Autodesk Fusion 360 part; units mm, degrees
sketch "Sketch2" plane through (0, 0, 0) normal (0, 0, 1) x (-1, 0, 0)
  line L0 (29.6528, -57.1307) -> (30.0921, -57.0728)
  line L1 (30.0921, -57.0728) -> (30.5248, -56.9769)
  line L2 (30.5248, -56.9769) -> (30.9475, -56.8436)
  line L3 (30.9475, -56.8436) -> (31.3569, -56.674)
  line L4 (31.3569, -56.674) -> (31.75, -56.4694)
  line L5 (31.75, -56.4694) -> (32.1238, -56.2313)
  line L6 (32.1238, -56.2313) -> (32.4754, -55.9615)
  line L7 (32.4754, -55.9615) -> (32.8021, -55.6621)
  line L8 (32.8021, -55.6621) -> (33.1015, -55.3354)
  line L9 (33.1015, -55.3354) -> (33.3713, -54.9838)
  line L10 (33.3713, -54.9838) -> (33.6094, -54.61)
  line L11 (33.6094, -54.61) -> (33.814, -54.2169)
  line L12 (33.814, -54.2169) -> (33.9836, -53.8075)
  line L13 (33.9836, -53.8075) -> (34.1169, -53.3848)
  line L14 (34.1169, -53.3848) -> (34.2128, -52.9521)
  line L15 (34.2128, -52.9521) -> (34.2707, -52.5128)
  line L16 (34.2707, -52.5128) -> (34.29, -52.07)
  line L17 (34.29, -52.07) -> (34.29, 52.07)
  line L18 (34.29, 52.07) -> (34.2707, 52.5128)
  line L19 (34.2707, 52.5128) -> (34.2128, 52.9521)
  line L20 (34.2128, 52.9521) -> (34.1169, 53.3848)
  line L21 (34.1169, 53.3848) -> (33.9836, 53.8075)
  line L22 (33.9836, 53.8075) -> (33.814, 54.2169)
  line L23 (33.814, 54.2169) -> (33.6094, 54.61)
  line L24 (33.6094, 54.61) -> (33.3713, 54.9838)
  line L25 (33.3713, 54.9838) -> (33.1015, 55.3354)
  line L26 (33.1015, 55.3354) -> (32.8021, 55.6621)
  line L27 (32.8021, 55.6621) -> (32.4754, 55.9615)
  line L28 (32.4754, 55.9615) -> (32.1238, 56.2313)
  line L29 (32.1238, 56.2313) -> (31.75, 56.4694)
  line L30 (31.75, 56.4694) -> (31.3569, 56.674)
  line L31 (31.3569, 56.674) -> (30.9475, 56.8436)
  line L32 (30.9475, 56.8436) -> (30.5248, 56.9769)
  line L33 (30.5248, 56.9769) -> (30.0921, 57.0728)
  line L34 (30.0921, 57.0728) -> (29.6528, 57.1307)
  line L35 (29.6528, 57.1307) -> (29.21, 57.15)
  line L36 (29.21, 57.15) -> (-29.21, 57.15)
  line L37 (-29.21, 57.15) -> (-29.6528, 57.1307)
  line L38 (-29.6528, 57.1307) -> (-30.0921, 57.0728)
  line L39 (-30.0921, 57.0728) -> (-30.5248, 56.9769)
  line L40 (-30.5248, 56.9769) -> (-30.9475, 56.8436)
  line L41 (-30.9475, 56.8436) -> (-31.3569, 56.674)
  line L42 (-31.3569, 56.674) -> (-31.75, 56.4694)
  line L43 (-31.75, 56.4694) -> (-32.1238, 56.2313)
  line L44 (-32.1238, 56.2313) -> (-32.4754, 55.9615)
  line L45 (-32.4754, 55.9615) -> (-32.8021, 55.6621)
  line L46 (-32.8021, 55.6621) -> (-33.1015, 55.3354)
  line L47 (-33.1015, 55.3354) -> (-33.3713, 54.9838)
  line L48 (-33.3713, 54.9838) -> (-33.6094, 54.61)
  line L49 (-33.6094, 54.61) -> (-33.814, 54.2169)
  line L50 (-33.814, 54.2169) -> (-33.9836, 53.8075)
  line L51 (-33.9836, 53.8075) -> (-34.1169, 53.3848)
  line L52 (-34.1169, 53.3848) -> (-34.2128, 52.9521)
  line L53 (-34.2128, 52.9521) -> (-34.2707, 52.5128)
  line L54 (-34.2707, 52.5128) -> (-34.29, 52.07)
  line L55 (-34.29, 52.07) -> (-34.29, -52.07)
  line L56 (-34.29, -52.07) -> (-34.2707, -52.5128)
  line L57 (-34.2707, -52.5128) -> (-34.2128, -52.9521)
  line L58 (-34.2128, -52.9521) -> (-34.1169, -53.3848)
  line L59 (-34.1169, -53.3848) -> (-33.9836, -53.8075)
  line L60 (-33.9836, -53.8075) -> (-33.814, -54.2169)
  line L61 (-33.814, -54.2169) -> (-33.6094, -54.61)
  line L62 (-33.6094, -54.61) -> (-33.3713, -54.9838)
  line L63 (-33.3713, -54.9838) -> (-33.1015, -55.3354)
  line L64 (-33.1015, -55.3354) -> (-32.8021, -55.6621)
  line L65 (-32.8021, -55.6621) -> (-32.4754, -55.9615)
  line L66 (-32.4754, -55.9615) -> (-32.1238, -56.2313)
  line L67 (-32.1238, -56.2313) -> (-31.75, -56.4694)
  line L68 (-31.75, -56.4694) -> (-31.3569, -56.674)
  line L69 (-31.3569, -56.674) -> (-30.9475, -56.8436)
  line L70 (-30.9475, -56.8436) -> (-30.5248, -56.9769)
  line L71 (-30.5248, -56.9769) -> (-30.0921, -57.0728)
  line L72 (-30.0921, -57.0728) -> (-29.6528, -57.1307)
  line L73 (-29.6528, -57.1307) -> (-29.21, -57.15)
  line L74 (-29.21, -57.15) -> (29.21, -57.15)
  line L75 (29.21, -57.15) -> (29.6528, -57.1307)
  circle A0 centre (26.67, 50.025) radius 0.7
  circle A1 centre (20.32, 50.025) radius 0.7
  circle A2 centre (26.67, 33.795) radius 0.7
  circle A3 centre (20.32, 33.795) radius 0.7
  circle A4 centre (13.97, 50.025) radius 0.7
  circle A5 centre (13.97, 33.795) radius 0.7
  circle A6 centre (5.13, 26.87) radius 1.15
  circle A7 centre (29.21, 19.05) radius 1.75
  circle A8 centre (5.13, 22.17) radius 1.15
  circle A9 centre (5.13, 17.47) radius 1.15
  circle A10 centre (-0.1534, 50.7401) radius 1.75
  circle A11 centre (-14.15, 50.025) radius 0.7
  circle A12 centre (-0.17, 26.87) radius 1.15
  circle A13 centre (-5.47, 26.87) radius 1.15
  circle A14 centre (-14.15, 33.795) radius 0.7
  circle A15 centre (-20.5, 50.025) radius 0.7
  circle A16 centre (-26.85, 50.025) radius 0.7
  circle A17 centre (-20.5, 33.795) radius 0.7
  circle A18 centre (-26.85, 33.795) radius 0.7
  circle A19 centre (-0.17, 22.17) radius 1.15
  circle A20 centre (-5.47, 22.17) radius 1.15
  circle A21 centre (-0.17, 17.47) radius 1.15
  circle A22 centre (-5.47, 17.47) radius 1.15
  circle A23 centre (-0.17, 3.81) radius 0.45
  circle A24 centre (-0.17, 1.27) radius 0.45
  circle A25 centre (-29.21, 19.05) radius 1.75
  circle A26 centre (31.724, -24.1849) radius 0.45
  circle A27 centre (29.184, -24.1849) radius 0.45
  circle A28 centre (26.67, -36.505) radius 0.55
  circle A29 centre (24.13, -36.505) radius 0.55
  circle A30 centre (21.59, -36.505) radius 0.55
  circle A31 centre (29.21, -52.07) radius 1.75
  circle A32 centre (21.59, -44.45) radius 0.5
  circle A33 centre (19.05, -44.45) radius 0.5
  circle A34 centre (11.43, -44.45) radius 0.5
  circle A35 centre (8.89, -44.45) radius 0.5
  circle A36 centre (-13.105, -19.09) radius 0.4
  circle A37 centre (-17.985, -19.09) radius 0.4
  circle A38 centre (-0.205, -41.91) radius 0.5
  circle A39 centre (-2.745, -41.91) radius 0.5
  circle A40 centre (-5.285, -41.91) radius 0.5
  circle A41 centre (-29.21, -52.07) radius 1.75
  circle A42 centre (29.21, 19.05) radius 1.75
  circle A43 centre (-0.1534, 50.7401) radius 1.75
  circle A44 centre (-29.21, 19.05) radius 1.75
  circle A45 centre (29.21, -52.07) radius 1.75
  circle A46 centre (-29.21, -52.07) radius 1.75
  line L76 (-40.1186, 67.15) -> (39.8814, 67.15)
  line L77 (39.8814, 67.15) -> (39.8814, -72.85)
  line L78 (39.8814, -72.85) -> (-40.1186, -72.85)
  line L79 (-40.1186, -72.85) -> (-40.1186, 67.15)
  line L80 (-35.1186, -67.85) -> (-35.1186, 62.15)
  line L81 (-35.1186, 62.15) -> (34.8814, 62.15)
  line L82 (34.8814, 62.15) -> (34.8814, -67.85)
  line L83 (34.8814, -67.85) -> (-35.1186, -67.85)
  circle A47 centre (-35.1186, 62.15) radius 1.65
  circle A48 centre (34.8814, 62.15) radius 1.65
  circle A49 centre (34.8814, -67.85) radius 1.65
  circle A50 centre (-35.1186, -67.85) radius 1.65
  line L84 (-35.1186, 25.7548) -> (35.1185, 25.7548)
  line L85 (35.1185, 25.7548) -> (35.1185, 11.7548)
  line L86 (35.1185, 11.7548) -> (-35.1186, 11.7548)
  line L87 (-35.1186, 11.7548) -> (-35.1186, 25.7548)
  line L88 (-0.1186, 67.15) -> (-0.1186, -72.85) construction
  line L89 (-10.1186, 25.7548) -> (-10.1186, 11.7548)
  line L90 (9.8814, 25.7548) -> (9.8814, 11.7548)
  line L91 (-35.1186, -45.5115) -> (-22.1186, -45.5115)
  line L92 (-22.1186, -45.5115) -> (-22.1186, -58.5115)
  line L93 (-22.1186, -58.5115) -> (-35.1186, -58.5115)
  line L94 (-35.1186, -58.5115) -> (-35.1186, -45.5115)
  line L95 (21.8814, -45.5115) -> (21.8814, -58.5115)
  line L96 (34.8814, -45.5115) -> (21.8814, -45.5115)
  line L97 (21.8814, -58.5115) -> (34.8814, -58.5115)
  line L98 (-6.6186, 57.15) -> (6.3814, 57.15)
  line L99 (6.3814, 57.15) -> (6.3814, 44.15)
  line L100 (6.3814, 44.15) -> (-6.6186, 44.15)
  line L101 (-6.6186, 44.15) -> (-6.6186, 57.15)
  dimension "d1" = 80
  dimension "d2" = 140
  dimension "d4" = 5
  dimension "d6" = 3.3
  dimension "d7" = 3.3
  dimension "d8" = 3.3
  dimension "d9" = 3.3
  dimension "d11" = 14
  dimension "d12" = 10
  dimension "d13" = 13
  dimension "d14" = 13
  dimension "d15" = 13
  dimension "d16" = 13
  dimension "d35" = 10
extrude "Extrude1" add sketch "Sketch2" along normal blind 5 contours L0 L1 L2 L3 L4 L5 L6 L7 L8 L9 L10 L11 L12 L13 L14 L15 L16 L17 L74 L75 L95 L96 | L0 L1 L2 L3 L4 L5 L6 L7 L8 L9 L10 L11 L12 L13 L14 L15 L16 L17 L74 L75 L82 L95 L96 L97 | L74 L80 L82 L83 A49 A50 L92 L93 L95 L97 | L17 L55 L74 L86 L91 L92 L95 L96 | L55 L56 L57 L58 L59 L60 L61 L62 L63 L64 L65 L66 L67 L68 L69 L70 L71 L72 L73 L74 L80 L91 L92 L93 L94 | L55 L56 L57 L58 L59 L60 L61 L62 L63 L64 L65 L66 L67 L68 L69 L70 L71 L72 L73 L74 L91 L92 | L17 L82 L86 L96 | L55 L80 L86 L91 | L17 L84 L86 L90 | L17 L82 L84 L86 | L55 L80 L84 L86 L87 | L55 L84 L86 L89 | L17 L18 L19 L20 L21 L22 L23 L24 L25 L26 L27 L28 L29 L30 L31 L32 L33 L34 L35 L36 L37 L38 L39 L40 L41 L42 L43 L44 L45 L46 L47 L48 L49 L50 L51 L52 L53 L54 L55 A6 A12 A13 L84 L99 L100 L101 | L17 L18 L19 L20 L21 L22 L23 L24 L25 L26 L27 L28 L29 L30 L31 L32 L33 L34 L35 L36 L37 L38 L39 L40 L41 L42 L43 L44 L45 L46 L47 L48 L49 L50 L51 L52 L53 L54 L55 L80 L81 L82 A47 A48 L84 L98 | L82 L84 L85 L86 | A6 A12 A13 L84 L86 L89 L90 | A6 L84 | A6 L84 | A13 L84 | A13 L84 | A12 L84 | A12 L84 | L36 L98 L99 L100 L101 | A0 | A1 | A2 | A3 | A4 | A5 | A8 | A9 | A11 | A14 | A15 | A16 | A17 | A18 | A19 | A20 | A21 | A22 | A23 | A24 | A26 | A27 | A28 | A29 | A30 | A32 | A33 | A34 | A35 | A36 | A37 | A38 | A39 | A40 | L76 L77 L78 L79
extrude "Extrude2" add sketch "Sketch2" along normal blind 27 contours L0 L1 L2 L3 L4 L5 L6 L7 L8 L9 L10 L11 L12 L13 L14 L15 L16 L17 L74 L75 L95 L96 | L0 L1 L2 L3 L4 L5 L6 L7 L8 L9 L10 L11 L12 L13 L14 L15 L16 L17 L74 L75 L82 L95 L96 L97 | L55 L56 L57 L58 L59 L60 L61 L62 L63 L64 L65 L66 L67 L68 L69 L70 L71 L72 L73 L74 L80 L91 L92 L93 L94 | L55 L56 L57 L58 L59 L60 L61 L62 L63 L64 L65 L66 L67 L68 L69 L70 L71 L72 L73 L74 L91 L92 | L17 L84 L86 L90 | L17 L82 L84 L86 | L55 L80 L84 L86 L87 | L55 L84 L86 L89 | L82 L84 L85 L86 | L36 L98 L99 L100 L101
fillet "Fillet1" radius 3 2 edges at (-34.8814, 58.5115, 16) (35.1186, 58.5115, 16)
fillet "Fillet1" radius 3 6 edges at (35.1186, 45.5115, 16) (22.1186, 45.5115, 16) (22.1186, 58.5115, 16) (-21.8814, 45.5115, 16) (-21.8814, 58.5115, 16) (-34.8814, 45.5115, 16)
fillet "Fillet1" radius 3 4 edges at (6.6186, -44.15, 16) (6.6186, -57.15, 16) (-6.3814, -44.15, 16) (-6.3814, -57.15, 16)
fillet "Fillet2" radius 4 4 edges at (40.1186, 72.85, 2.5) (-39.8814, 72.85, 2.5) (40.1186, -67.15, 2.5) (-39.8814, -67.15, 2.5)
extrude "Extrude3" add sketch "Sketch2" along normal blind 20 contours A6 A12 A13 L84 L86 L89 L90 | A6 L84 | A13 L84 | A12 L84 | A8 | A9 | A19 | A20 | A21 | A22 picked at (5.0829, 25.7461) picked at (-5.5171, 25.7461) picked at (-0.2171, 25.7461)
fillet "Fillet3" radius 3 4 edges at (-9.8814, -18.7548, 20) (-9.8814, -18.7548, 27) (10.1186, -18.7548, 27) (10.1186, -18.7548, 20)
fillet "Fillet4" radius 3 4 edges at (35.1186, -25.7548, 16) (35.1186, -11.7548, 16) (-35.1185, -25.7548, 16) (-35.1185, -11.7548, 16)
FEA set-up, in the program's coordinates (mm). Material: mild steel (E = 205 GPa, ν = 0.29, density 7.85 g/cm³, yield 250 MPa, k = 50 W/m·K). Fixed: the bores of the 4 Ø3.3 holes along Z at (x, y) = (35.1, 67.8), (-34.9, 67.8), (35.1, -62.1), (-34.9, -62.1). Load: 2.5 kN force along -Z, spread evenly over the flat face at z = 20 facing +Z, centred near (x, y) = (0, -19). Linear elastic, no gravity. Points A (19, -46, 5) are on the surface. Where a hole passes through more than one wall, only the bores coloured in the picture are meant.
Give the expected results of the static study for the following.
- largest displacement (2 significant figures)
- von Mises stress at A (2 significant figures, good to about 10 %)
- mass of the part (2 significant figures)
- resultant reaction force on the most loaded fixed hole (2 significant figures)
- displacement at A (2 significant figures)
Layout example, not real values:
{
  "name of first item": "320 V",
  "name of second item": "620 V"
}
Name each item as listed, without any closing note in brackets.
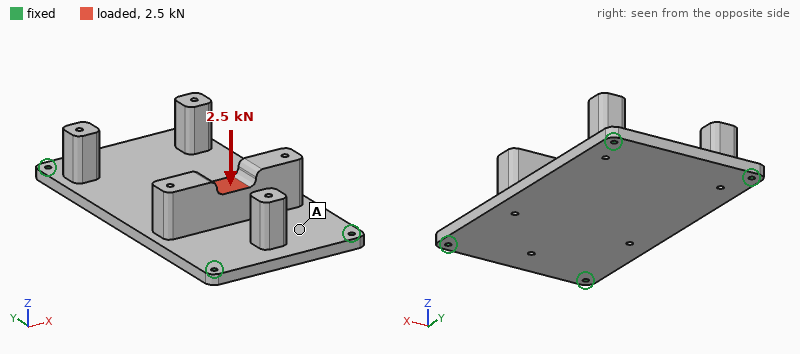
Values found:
{
  "largest displacement": "0.18 mm",
  "von Mises stress at A": "24 MPa",
  "mass of the part": "660 g",
  "resultant reaction force on the most loaded fixed hole": "880 N",
  "displacement at A": "0.064 mm"
}
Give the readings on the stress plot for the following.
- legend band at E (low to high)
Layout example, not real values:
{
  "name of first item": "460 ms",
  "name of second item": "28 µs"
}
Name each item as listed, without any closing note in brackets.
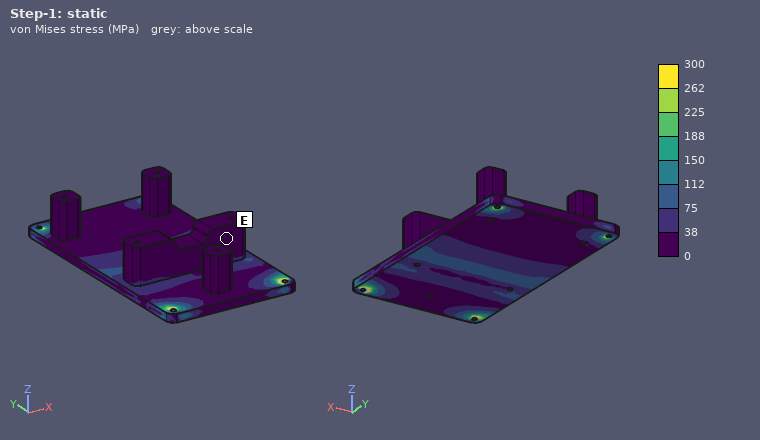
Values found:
{
  "legend band at E": "0 to 38 MPa"
}
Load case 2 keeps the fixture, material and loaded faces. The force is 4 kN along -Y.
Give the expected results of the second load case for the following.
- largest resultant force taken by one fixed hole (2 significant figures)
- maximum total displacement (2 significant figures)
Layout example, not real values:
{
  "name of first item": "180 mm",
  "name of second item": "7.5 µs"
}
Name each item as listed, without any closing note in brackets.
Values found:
{
  "largest resultant force taken by one fixed hole": "1.3 kN",
  "maximum total displacement": "0.12 mm"
}
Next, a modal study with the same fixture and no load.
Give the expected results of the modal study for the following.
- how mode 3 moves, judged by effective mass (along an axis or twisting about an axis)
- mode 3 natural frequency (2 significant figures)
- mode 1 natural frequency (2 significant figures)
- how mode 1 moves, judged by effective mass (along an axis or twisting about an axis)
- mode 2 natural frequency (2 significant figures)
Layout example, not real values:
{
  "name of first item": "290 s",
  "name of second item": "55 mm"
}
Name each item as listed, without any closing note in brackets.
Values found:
{
  "how mode 3 moves, judged by effective mass": "twisting about X",
  "mode 3 natural frequency": "2700 Hz",
  "mode 1 natural frequency": "980 Hz",
  "how mode 1 moves, judged by effective mass": "along Z",
  "mode 2 natural frequency": "1900 Hz"
}
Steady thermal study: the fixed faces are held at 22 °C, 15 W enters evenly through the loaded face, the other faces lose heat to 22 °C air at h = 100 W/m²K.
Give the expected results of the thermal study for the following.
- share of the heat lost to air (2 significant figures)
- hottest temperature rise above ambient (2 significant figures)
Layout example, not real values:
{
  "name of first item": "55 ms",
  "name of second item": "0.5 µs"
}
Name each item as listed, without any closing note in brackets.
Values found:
{
  "share of the heat lost to air": "85 %",
  "hottest temperature rise above ambient": "22 K"
}
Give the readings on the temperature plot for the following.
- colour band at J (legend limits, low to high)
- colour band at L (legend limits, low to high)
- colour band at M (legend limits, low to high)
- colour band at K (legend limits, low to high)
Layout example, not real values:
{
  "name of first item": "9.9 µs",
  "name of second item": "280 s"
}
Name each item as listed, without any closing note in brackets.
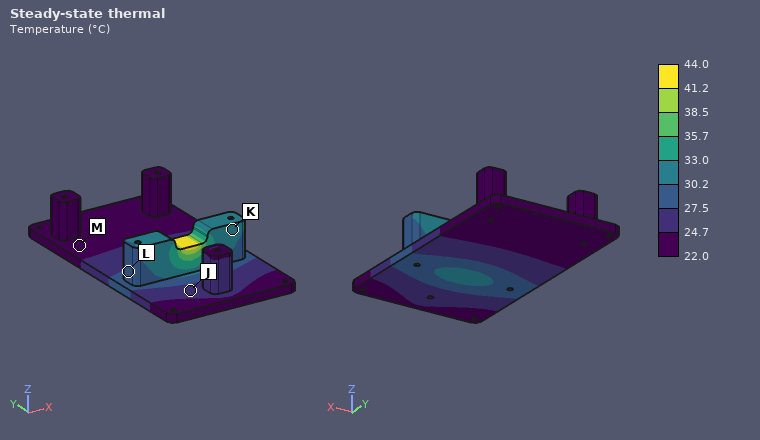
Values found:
{
  "colour band at J": "24.7 to 27.5 °C",
  "colour band at L": "27.5 to 30.2 °C",
  "colour band at M": "22.0 to 24.7 °C",
  "colour band at K": "30.2 to 33.0 °C"
}
